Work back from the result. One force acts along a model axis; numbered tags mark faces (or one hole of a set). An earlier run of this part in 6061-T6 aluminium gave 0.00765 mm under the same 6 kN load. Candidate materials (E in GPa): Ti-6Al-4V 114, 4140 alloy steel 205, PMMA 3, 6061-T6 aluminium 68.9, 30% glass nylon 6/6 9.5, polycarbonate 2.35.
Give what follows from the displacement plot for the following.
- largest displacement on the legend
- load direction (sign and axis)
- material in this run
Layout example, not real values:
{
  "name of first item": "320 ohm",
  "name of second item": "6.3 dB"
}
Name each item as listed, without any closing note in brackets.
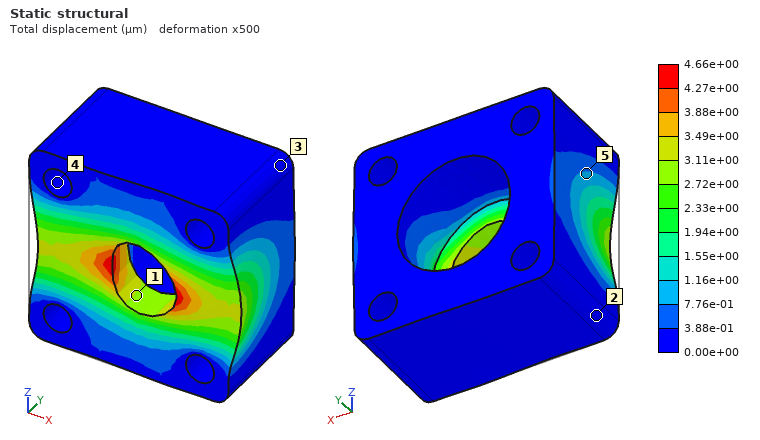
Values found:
{
  "largest displacement on the legend": "4.66e+00 µm",
  "load direction": "+X",
  "material in this run": "Ti-6Al-4V"
}
